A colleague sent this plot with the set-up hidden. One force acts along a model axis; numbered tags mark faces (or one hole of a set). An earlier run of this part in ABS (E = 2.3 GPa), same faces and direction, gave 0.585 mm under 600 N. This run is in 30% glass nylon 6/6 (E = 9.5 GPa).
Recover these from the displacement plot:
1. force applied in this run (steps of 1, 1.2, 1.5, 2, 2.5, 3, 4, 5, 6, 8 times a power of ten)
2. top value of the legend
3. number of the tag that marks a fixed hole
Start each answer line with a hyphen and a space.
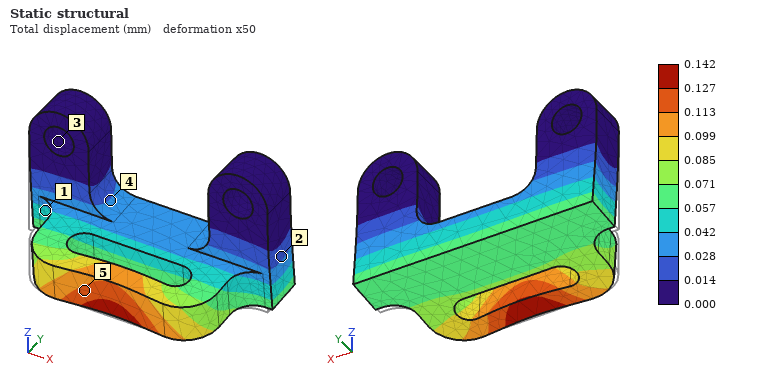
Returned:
- 600 N
- 0.142 mm
- 3
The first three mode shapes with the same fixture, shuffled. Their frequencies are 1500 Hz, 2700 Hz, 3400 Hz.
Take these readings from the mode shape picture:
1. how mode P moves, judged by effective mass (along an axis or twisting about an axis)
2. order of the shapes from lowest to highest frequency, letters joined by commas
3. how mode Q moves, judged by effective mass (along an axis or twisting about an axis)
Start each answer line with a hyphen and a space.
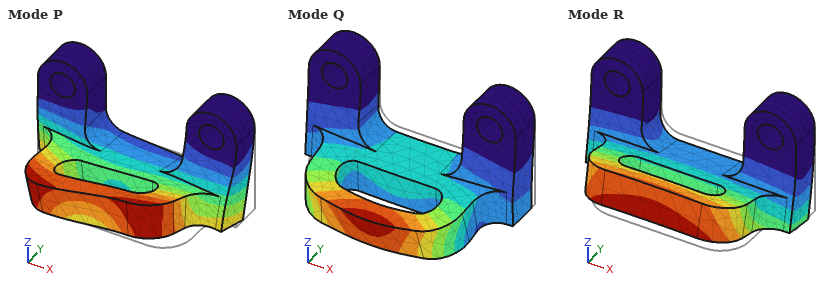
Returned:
- along X
- R, P, Q
- along Y
